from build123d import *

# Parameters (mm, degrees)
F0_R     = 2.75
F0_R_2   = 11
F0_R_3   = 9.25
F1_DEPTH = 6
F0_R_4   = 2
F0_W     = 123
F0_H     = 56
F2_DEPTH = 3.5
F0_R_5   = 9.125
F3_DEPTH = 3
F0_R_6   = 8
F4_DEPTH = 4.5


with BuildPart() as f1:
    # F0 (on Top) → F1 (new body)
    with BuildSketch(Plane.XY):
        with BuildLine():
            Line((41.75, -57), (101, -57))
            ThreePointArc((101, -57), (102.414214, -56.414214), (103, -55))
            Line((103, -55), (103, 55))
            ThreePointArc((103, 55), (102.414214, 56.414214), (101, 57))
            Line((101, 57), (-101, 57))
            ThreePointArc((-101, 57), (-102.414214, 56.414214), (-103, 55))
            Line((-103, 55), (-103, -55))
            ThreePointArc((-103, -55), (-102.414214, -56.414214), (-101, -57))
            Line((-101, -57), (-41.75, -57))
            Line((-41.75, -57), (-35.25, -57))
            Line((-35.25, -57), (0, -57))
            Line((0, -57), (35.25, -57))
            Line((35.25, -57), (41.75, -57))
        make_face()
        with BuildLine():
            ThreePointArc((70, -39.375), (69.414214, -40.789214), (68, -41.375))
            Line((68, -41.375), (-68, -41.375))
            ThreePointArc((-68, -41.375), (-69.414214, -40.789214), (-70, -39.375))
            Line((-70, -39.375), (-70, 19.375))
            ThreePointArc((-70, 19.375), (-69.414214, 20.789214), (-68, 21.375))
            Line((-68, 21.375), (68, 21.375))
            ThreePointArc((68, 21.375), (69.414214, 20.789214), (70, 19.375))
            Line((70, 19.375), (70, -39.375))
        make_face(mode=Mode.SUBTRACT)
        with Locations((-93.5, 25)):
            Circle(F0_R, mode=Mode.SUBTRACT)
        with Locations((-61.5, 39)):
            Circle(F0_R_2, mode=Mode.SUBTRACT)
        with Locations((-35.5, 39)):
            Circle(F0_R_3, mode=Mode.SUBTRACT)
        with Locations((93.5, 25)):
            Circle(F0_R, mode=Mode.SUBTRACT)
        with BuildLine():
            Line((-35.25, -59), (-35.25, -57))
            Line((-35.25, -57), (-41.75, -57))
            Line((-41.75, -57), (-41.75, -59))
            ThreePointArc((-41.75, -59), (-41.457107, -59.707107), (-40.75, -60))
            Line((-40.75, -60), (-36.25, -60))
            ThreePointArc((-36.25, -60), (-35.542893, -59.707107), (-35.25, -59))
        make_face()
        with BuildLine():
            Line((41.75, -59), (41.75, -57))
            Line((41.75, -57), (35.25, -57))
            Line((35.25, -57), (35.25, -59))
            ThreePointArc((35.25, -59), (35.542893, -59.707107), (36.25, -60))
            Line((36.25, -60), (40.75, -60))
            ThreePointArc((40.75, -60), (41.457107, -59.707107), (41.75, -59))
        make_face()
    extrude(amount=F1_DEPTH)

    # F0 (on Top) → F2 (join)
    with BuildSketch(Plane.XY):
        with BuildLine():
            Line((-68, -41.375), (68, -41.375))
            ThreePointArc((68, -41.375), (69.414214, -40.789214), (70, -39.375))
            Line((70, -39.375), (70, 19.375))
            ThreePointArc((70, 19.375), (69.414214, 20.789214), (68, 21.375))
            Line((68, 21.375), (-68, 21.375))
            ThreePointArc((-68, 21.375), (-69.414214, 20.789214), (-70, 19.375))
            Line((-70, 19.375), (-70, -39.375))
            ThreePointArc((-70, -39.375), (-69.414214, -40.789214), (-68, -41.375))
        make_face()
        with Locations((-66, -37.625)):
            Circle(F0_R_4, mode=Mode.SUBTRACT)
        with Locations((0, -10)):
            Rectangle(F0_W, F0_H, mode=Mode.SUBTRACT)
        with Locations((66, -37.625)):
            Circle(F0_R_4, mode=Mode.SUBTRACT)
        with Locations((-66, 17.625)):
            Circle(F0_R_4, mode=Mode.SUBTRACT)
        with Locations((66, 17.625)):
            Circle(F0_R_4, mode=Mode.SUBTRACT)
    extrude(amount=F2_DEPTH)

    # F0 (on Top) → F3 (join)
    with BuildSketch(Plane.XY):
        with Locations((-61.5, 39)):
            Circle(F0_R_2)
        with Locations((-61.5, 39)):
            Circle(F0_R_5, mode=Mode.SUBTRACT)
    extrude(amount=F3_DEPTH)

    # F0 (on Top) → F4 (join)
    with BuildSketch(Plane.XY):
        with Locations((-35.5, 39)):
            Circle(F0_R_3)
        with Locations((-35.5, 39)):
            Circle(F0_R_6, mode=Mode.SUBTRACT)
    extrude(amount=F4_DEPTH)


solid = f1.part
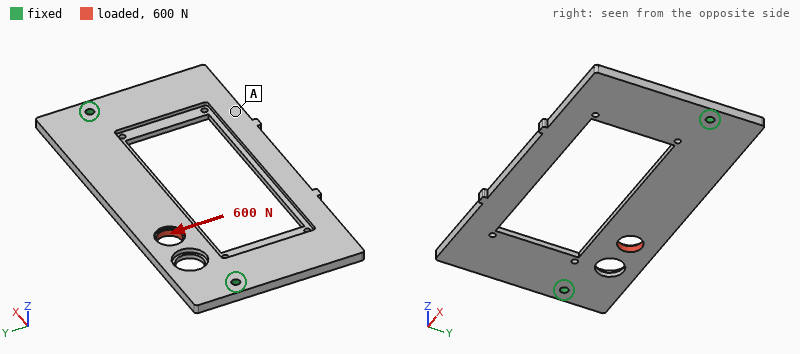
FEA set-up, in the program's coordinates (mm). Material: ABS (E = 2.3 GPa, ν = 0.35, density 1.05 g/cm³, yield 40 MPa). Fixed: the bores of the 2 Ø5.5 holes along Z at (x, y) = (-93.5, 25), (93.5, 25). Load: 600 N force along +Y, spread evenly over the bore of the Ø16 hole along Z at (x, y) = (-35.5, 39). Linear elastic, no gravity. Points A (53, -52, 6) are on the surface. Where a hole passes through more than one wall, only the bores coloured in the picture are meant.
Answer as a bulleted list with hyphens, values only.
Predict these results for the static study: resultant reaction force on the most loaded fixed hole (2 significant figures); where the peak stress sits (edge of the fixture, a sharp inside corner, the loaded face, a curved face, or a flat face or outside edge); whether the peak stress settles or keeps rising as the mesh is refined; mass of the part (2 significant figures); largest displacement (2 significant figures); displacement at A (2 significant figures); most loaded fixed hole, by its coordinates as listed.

- 440 N
- a sharp inside corner
- keeps rising
- 96 g
- 0.57 mm
- 0.29 mm
- (-93.5, 25)
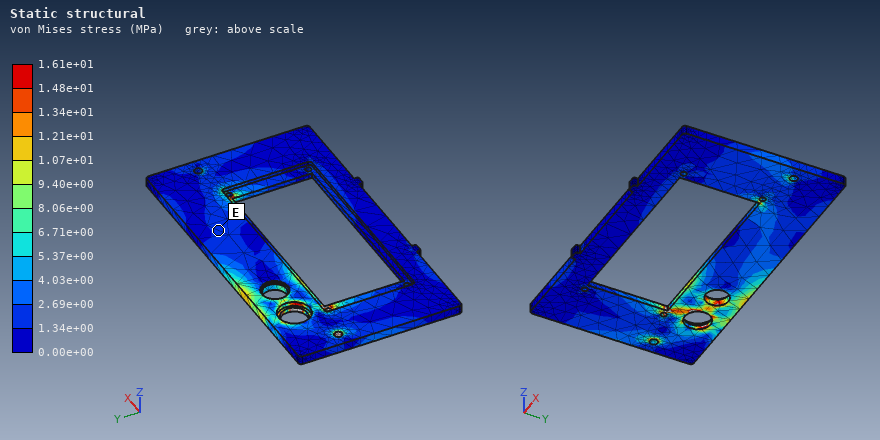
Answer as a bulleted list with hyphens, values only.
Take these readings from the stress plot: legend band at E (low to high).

- 1.34e+00 to 2.69e+00 MPa
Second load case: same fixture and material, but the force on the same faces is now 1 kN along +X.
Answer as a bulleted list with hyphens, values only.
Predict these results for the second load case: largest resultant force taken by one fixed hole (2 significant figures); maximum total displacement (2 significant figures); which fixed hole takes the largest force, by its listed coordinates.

- 560 N
- 0.25 mm
- (-93.5, 25)
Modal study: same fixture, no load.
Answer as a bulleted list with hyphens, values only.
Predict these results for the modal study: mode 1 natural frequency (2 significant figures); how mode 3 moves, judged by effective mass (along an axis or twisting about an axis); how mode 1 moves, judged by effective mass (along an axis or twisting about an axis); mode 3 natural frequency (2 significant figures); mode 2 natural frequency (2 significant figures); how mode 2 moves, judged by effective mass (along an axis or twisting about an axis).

- 120 Hz
- along Z
- along Z
- 250 Hz
- 220 Hz
- twisting about Y
